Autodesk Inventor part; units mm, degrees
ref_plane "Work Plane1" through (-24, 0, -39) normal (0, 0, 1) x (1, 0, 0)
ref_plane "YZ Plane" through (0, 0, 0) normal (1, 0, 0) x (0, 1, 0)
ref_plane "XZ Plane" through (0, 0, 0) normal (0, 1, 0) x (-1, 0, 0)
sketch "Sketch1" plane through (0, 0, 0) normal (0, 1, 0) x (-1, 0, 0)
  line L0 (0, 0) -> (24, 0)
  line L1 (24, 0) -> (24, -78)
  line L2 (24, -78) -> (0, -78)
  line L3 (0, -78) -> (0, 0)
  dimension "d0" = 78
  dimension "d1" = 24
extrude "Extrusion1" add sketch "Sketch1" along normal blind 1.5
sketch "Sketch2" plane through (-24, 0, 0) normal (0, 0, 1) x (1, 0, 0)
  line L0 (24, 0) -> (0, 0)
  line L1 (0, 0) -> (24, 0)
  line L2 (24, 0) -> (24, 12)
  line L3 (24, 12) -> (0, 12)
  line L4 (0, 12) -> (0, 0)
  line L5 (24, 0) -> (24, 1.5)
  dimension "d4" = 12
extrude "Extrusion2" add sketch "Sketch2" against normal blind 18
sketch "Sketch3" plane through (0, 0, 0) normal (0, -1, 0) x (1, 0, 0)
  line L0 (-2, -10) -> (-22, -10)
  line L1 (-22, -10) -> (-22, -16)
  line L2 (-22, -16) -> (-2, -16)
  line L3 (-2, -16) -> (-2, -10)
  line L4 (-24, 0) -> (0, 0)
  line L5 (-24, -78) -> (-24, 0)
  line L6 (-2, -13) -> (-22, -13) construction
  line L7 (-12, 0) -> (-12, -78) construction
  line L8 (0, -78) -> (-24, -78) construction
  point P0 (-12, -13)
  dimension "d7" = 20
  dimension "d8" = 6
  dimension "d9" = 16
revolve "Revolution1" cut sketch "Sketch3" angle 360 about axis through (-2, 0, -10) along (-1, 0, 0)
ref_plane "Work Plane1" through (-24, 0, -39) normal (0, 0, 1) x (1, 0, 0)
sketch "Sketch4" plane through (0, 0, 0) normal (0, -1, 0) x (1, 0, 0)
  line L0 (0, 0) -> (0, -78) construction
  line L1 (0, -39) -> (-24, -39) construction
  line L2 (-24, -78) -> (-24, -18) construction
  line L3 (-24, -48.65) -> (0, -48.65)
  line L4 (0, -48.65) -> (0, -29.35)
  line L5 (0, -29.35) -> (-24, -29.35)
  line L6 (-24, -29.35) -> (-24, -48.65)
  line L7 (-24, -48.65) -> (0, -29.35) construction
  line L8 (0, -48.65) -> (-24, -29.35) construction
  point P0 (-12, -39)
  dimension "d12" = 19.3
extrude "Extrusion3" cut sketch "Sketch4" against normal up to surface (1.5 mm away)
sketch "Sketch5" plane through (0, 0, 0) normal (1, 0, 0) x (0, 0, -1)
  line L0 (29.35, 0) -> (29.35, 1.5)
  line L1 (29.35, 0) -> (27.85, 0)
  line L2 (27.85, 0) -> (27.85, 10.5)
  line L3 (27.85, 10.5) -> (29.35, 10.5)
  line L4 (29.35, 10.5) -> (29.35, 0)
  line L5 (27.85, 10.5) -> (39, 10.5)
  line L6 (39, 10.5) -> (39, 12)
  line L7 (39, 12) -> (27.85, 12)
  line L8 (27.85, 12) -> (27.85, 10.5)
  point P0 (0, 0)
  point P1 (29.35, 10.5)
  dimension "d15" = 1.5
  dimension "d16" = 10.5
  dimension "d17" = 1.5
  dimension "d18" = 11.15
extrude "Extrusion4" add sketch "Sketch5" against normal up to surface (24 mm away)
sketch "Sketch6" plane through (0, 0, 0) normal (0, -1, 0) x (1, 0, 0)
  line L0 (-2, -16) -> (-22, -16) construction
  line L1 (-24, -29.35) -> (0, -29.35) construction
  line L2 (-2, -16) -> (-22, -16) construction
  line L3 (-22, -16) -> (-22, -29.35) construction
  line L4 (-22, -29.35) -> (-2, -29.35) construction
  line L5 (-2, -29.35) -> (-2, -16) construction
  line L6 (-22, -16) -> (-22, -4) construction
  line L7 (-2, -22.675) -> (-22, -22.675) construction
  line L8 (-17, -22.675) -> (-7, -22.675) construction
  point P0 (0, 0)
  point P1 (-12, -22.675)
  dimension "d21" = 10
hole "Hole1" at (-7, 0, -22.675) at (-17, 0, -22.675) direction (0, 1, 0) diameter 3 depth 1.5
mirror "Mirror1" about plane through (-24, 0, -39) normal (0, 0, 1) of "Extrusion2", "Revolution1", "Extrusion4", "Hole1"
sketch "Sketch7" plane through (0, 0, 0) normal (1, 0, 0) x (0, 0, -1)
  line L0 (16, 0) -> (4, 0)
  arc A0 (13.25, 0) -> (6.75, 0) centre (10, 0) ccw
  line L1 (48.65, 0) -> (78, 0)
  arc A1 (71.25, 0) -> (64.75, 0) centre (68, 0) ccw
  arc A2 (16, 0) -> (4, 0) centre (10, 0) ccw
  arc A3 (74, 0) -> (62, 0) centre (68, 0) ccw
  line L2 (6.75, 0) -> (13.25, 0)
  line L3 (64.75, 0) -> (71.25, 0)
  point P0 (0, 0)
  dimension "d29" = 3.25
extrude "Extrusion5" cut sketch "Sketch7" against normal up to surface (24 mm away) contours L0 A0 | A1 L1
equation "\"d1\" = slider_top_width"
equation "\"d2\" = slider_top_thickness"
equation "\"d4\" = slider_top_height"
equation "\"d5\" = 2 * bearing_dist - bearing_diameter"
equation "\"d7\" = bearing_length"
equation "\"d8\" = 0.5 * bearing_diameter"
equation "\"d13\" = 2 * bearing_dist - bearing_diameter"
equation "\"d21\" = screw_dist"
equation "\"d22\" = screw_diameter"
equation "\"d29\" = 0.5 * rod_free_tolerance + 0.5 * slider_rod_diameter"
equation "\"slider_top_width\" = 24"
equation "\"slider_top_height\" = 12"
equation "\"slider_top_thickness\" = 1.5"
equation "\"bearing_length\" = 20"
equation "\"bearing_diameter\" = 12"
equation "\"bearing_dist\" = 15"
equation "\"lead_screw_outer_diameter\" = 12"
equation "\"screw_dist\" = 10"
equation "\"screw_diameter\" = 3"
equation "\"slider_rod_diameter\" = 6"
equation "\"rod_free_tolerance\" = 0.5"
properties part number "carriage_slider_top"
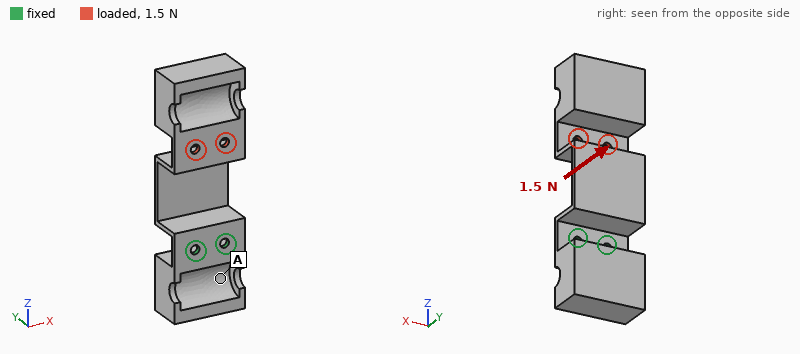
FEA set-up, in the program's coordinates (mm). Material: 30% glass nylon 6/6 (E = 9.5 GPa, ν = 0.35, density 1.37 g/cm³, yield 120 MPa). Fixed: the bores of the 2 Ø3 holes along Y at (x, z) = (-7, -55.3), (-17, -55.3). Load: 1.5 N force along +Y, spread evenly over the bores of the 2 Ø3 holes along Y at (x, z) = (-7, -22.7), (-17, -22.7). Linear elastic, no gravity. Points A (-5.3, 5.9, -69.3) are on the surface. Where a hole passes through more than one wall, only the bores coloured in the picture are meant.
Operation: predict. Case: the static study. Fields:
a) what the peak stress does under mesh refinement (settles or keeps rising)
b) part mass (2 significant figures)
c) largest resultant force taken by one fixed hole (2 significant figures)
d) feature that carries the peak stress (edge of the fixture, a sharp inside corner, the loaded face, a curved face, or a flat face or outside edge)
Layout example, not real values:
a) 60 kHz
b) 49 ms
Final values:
a) keeps rising
b) 14 g
c) 0.75 N
d) edge of the fixture
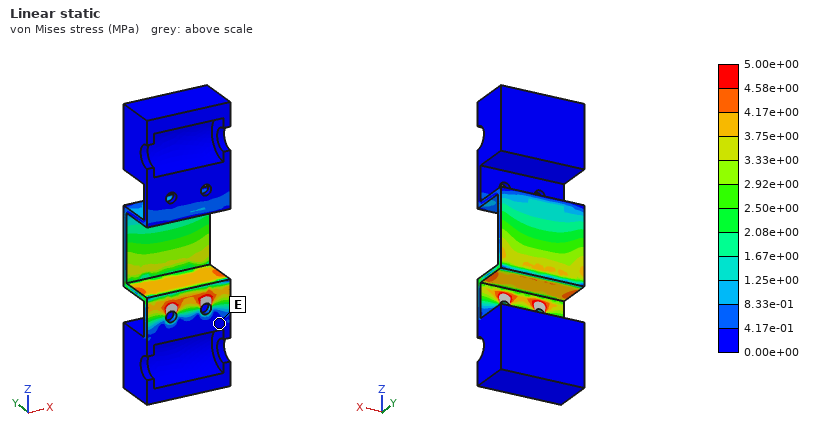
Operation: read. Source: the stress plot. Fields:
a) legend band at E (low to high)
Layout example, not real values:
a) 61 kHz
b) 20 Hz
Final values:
a) 0.00e+00 to 4.17e-01 MPa
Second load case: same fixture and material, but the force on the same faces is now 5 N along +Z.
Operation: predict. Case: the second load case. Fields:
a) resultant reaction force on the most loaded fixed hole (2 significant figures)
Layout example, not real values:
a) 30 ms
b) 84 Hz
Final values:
a) 2.5 N
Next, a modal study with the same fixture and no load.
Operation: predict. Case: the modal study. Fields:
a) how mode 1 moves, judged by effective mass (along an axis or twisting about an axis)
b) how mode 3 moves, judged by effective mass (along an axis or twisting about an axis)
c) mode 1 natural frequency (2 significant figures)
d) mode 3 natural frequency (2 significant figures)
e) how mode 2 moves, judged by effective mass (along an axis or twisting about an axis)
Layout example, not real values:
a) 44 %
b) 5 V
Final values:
a) along Y
b) along Z
c) 76 Hz
d) 470 Hz
e) along X
